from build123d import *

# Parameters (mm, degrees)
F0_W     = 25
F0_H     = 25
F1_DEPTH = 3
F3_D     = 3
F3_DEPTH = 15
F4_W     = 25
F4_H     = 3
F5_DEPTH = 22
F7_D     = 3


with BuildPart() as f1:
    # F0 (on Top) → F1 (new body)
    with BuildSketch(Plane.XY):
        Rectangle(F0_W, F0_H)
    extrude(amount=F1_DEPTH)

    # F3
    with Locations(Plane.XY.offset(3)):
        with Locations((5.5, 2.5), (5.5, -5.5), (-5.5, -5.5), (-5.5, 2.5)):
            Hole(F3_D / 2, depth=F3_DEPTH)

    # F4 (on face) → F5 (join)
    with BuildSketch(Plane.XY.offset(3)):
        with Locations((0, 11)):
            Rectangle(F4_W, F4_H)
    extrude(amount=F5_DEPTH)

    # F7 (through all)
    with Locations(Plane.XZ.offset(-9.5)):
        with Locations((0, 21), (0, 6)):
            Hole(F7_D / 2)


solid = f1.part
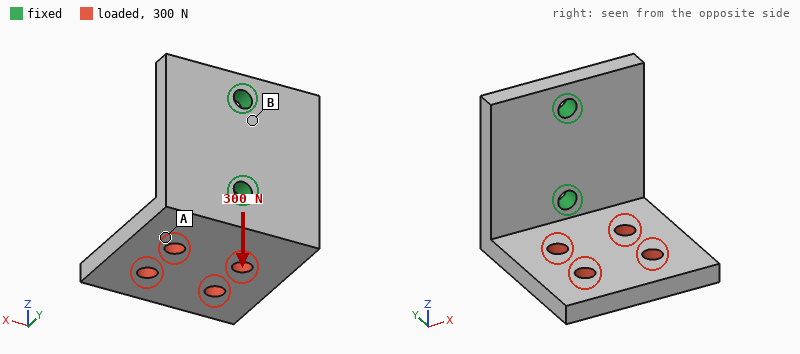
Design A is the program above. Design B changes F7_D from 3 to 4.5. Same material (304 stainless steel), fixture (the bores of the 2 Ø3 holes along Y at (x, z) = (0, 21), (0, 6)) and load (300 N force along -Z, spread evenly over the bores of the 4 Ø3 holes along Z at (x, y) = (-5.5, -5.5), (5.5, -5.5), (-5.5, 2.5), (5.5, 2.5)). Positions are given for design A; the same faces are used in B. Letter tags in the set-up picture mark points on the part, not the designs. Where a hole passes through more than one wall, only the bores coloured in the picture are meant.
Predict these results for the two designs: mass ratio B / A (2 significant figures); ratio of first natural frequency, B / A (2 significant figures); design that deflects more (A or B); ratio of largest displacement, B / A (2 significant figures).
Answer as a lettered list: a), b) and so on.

a) 0.98
b) 1.1
c) A
d) 0.88
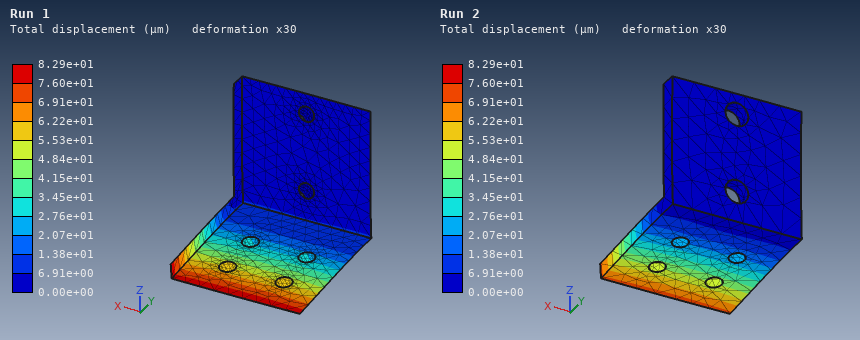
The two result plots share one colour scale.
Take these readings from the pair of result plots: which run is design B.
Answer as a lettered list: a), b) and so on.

a) Run 2
